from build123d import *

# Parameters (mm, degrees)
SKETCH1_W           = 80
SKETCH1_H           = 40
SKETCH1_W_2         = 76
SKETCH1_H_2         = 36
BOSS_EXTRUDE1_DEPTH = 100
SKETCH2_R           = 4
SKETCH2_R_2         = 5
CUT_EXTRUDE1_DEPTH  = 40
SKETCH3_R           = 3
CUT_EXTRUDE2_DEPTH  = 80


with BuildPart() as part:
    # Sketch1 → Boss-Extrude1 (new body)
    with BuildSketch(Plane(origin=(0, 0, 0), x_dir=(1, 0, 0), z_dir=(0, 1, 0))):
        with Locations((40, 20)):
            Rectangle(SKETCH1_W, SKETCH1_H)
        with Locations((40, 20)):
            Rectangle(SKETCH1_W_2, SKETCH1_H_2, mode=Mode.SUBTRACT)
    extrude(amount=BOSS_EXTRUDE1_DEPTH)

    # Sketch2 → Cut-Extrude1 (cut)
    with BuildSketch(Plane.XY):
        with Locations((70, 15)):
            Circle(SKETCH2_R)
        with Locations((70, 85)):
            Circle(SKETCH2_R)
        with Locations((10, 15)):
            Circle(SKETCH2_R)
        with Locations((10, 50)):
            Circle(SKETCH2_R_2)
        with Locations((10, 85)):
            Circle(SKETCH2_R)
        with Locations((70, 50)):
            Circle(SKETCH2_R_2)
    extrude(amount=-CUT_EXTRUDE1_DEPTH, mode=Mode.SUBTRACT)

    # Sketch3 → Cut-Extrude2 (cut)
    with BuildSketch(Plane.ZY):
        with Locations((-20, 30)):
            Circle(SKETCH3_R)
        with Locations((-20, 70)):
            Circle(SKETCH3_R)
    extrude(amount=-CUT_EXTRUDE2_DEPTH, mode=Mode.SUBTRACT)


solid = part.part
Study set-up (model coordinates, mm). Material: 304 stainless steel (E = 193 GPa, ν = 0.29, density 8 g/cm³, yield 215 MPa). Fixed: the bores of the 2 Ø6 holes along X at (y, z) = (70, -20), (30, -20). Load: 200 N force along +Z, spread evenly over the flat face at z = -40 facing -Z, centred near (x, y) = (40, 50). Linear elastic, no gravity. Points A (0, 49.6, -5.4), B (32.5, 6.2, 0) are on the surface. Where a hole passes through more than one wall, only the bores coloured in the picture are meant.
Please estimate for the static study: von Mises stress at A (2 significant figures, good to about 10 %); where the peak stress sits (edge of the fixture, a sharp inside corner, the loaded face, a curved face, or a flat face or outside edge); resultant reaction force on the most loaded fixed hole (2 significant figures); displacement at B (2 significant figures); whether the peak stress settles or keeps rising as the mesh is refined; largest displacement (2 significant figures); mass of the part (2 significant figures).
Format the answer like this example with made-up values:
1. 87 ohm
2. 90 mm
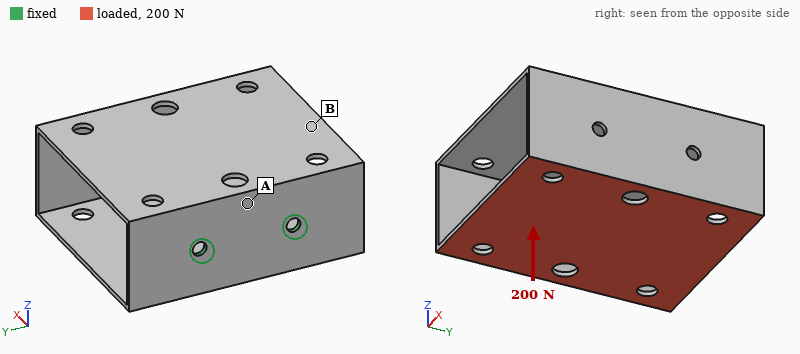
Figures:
1. 31 MPa
2. edge of the fixture
3. 100 N
4. 0.21 mm
5. keeps rising
6. 0.53 mm
7. 360 g
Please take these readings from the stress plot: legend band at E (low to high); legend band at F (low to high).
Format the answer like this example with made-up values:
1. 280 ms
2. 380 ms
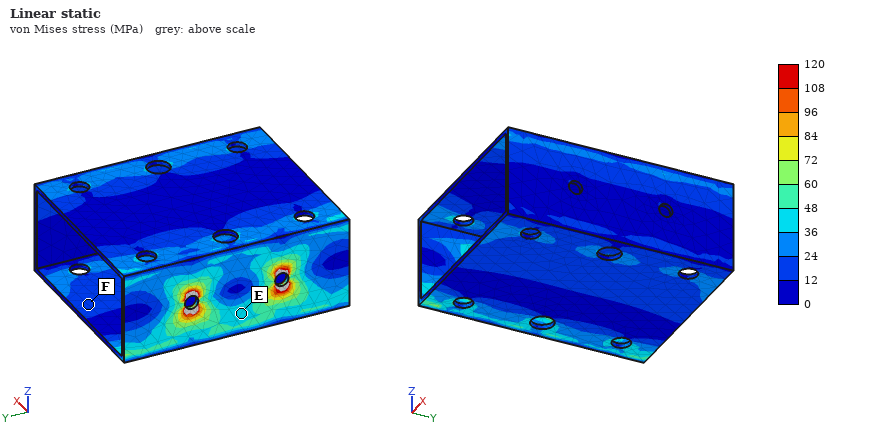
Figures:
1. 36 to 48 MPa
2. 12 to 24 MPa
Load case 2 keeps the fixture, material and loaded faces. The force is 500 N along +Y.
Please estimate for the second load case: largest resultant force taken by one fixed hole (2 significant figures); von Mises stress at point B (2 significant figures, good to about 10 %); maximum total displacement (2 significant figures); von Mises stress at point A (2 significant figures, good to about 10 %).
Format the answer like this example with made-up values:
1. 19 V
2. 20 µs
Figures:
1. 520 N
2. 11 MPa
3. 0.24 mm
4. 26 MPa
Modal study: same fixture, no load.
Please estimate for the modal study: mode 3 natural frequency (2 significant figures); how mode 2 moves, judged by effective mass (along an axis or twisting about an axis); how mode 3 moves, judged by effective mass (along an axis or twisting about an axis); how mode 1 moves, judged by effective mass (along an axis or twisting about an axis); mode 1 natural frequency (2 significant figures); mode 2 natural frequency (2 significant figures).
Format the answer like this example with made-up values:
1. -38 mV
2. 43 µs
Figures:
1. 620 Hz
2. along Y
3. twisting about X
4. along Z
5. 180 Hz
6. 480 Hz
